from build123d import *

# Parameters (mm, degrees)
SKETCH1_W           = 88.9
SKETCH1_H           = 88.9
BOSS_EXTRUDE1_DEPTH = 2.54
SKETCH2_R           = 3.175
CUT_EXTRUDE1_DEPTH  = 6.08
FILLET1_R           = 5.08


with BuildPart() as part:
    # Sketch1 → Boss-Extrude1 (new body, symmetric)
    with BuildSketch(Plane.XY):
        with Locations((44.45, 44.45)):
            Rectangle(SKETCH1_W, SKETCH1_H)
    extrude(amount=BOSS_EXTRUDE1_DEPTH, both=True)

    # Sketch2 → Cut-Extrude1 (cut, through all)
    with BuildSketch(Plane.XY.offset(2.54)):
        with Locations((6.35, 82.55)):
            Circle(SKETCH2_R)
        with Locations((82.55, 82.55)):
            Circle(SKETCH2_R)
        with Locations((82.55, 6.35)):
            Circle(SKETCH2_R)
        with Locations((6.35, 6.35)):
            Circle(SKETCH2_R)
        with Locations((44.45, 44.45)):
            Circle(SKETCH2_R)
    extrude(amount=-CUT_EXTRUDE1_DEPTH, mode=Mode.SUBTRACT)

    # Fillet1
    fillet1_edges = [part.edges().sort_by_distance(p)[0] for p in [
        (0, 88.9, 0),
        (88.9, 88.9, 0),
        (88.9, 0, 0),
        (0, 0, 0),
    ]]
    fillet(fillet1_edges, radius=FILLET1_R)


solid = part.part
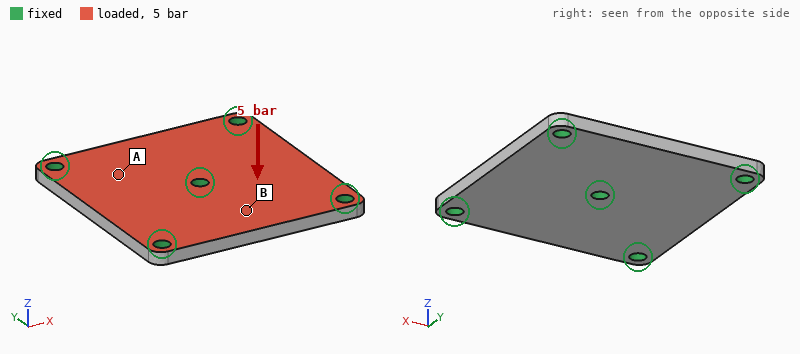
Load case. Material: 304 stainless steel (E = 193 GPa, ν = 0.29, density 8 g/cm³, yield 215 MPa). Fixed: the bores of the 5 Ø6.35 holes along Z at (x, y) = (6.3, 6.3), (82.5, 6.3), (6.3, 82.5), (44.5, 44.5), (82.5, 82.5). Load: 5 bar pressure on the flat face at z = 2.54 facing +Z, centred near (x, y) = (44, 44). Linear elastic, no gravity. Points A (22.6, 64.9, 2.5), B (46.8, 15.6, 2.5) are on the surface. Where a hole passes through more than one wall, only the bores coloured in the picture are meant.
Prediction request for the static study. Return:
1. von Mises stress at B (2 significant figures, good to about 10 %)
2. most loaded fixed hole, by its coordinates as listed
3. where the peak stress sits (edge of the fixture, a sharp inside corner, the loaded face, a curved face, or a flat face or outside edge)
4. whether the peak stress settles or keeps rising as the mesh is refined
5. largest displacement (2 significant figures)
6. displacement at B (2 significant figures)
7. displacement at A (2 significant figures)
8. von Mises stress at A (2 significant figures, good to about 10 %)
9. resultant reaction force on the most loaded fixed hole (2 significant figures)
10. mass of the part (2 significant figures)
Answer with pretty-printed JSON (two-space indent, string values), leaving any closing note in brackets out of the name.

{
  "von Mises stress at B": "8.5 MPa",
  "most loaded fixed hole, by its coordinates as listed": "(44.5, 44.5)",
  "where the peak stress sits": "edge of the fixture",
  "whether the peak stress settles or keeps rising as the mesh is refined": "keeps rising",
  "largest displacement": "14 µm",
  "displacement at B": "10.0 µm",
  "displacement at A": "7.4 µm",
  "von Mises stress at A": "20 MPa",
  "resultant reaction force on the most loaded fixed hole": "1.5 kN",
  "mass of the part": "310 g"
}
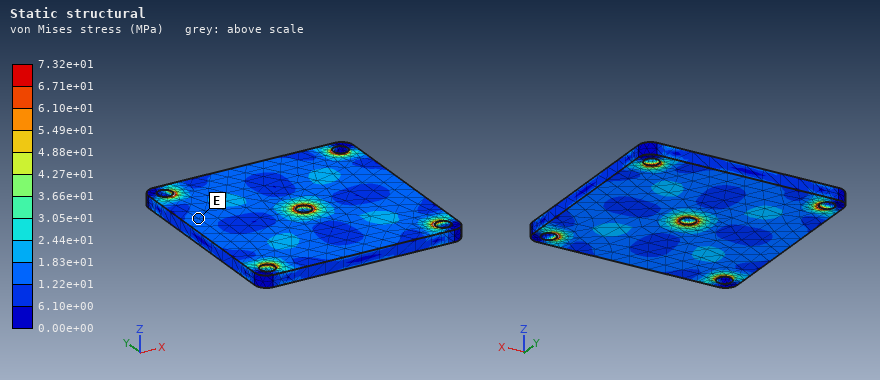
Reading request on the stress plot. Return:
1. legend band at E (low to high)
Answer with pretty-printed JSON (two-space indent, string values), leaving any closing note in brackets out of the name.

{
  "legend band at E": "1.22e+01 to 1.83e+01 MPa"
}
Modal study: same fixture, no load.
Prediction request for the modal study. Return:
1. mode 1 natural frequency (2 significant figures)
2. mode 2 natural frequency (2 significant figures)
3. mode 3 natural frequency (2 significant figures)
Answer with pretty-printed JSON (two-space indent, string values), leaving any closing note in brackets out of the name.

{
  "mode 1 natural frequency": "5500 Hz",
  "mode 2 natural frequency": "5600 Hz",
  "mode 3 natural frequency": "5600 Hz"
}
